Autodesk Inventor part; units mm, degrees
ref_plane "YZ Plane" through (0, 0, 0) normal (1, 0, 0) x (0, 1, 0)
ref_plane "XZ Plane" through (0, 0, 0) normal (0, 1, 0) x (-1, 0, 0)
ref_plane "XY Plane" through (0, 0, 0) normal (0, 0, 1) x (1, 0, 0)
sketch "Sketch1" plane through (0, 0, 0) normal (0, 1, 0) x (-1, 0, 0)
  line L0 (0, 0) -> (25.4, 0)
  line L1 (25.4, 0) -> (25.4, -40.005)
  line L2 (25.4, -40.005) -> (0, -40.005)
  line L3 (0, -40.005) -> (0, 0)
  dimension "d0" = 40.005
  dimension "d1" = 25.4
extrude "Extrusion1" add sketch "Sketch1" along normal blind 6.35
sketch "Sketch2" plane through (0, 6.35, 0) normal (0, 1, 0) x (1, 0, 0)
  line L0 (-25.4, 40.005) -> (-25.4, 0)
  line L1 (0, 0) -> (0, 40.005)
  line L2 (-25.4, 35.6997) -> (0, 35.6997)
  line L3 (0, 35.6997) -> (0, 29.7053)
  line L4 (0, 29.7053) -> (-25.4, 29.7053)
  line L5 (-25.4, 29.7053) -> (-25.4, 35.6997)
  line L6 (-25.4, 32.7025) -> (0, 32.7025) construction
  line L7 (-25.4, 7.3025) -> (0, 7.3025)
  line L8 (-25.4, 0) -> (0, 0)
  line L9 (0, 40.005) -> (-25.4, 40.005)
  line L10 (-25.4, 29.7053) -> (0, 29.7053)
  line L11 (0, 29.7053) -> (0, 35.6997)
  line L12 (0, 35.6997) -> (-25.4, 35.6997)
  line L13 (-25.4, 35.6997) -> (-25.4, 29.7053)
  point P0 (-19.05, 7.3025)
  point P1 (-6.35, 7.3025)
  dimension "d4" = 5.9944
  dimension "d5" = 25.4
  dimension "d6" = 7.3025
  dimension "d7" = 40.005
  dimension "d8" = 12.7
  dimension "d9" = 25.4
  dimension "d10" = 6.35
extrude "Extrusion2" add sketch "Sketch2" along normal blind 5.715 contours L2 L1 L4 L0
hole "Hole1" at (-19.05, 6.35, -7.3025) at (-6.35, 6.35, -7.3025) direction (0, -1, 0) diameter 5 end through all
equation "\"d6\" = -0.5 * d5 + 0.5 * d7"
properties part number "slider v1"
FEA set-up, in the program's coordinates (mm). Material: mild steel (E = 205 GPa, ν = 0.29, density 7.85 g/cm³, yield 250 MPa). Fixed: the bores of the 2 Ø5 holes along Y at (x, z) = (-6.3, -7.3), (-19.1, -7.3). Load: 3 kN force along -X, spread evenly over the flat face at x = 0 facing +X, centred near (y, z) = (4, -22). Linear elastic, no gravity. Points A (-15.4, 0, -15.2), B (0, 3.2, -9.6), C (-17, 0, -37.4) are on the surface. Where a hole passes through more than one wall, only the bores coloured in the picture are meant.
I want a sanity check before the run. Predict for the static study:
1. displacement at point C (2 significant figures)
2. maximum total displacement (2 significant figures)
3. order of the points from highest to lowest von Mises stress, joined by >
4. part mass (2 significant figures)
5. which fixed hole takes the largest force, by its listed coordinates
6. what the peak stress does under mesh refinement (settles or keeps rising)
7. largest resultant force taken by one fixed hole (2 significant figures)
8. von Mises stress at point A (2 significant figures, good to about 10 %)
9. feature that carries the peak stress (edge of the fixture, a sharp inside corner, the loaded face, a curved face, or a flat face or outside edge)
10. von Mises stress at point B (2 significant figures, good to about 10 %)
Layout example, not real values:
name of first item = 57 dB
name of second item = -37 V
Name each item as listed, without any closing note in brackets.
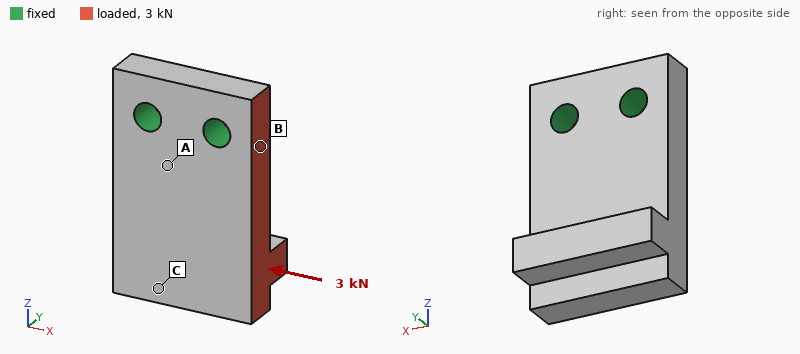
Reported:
displacement at point C = 9.9 µm
maximum total displacement = 14 µm
order of the points from highest to lowest von Mises stress, joined by > = B > A > C
part mass = 56 g
which fixed hole takes the largest force, by its listed coordinates = (-6.3, -7.3)
what the peak stress does under mesh refinement = keeps rising
largest resultant force taken by one fixed hole = 3.1 kN
von Mises stress at point A = 29 MPa
feature that carries the peak stress = edge of the fixture
von Mises stress at point B = 51 MPa
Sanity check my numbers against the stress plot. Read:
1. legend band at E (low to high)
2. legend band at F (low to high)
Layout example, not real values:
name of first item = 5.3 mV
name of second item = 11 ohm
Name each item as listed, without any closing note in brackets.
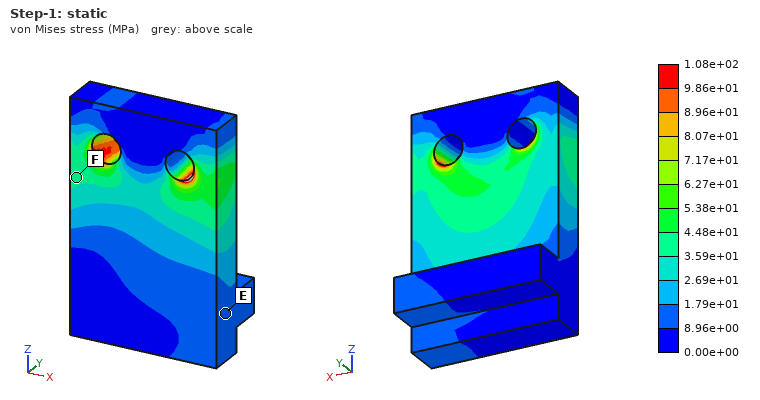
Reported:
legend band at E = 8.96e+00 to 1.79e+01 MPa
legend band at F = 3.59e+01 to 4.48e+01 MPa
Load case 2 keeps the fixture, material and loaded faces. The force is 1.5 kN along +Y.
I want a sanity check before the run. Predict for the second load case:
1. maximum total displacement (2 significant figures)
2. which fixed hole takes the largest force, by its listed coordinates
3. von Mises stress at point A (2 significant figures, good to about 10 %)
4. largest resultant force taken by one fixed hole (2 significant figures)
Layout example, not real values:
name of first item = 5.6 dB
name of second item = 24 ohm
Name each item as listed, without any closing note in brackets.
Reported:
maximum total displacement = 65 µm
which fixed hole takes the largest force, by its listed coordinates = (-6.3, -7.3)
von Mises stress at point A = 79 MPa
largest resultant force taken by one fixed hole = 1.7 kN
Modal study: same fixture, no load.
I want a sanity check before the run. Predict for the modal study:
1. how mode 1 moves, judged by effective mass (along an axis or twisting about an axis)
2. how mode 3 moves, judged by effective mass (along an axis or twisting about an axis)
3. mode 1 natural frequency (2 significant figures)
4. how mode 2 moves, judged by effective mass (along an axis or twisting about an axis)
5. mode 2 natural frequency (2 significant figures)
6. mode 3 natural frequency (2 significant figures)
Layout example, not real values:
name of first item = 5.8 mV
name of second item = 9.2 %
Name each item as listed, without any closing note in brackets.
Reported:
how mode 1 moves, judged by effective mass = along Y
how mode 3 moves, judged by effective mass = along X
mode 1 natural frequency = 4400 Hz
how mode 2 moves, judged by effective mass = along X
mode 2 natural frequency = 11 kHz
mode 3 natural frequency = 13 kHz
